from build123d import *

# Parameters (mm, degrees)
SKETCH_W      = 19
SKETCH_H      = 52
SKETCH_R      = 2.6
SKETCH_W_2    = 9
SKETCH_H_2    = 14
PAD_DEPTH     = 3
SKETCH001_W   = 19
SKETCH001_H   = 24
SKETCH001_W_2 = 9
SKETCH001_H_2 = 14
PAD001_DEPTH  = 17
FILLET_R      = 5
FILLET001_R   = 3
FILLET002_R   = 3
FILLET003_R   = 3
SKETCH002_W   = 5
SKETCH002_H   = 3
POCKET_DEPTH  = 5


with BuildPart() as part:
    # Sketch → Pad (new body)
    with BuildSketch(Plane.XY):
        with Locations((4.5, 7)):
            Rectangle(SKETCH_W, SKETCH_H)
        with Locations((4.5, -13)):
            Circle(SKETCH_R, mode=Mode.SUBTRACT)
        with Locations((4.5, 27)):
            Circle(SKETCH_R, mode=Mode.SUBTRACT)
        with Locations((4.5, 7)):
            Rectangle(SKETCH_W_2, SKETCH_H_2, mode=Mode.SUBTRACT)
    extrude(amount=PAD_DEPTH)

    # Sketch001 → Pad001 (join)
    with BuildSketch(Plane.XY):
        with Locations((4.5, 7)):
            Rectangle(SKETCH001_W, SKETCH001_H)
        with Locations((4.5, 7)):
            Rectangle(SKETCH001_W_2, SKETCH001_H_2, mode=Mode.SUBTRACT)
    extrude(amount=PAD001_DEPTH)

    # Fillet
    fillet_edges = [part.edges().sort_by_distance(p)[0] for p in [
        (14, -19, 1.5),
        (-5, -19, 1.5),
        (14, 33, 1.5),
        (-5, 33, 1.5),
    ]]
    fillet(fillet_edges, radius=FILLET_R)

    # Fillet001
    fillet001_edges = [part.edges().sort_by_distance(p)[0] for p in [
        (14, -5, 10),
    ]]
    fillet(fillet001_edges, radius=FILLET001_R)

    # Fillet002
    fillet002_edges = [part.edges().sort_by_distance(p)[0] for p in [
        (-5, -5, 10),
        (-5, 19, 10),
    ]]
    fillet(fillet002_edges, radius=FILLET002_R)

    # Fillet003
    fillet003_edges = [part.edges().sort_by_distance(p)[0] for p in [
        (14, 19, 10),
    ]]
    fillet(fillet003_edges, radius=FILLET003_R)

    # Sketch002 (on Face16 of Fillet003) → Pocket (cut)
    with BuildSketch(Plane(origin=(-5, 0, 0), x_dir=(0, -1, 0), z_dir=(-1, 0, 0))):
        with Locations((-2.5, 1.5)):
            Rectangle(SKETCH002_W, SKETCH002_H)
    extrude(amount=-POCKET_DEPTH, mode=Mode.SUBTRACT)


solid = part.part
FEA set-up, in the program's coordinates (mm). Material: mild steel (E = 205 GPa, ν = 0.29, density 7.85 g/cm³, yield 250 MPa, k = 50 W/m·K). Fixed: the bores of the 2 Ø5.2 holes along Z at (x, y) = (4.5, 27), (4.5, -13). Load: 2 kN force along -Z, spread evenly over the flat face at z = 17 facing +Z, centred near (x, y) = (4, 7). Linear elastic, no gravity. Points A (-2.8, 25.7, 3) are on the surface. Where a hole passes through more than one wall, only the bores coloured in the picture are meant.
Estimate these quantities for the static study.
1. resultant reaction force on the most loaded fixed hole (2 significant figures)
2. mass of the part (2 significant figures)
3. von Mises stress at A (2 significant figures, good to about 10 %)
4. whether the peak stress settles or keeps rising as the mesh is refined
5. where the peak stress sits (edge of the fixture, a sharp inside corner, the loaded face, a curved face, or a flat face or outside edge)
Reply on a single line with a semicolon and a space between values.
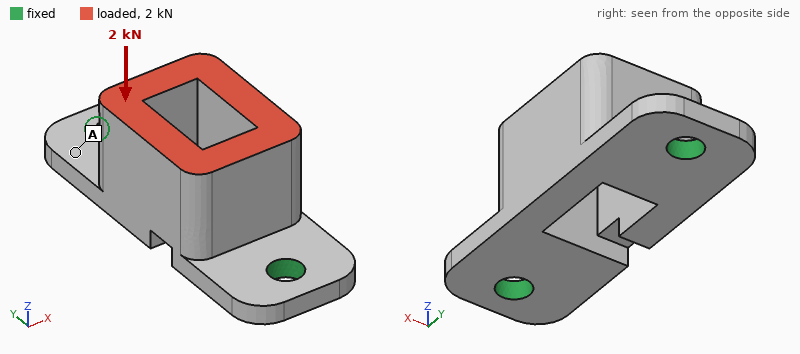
1.2 kN; 54 g; 32 MPa; keeps rising; edge of the fixture
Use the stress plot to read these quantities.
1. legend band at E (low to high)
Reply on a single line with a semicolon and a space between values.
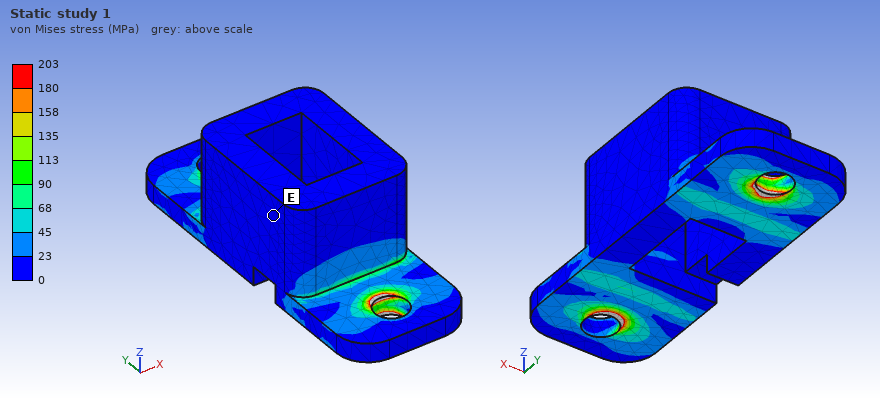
0 to 23 MPa
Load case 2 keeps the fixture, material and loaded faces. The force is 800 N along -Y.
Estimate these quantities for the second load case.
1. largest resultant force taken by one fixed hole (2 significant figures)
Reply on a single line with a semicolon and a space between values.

570 N
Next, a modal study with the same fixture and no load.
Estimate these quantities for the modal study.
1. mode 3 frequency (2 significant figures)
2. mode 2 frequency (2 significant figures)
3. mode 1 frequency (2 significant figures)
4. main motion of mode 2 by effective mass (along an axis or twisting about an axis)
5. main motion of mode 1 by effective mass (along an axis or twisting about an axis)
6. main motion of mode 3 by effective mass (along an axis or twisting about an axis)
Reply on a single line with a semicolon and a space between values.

14 kHz; 11 kHz; 4900 Hz; along Z; along X; along Y
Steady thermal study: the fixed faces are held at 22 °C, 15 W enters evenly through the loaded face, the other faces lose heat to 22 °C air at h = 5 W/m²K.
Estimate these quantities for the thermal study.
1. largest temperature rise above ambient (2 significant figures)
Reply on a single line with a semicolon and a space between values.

41 K
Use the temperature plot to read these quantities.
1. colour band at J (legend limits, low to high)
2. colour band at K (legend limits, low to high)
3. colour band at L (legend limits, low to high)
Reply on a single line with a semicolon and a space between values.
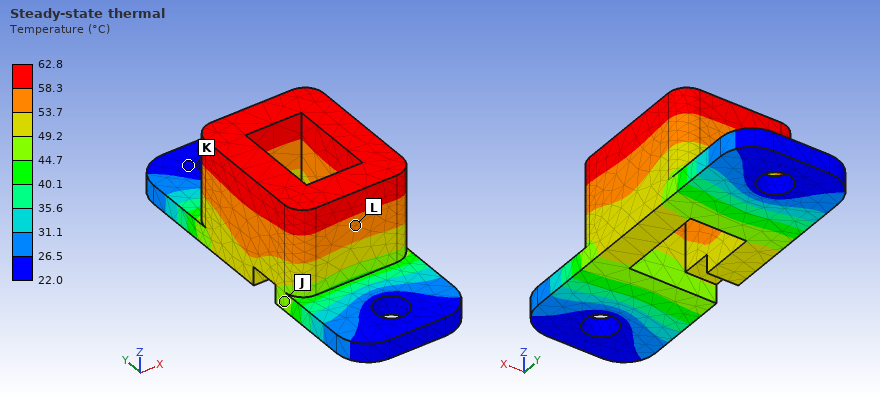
44.7 to 49.2 °C; 22.0 to 26.5 °C; 53.7 to 58.3 °C
